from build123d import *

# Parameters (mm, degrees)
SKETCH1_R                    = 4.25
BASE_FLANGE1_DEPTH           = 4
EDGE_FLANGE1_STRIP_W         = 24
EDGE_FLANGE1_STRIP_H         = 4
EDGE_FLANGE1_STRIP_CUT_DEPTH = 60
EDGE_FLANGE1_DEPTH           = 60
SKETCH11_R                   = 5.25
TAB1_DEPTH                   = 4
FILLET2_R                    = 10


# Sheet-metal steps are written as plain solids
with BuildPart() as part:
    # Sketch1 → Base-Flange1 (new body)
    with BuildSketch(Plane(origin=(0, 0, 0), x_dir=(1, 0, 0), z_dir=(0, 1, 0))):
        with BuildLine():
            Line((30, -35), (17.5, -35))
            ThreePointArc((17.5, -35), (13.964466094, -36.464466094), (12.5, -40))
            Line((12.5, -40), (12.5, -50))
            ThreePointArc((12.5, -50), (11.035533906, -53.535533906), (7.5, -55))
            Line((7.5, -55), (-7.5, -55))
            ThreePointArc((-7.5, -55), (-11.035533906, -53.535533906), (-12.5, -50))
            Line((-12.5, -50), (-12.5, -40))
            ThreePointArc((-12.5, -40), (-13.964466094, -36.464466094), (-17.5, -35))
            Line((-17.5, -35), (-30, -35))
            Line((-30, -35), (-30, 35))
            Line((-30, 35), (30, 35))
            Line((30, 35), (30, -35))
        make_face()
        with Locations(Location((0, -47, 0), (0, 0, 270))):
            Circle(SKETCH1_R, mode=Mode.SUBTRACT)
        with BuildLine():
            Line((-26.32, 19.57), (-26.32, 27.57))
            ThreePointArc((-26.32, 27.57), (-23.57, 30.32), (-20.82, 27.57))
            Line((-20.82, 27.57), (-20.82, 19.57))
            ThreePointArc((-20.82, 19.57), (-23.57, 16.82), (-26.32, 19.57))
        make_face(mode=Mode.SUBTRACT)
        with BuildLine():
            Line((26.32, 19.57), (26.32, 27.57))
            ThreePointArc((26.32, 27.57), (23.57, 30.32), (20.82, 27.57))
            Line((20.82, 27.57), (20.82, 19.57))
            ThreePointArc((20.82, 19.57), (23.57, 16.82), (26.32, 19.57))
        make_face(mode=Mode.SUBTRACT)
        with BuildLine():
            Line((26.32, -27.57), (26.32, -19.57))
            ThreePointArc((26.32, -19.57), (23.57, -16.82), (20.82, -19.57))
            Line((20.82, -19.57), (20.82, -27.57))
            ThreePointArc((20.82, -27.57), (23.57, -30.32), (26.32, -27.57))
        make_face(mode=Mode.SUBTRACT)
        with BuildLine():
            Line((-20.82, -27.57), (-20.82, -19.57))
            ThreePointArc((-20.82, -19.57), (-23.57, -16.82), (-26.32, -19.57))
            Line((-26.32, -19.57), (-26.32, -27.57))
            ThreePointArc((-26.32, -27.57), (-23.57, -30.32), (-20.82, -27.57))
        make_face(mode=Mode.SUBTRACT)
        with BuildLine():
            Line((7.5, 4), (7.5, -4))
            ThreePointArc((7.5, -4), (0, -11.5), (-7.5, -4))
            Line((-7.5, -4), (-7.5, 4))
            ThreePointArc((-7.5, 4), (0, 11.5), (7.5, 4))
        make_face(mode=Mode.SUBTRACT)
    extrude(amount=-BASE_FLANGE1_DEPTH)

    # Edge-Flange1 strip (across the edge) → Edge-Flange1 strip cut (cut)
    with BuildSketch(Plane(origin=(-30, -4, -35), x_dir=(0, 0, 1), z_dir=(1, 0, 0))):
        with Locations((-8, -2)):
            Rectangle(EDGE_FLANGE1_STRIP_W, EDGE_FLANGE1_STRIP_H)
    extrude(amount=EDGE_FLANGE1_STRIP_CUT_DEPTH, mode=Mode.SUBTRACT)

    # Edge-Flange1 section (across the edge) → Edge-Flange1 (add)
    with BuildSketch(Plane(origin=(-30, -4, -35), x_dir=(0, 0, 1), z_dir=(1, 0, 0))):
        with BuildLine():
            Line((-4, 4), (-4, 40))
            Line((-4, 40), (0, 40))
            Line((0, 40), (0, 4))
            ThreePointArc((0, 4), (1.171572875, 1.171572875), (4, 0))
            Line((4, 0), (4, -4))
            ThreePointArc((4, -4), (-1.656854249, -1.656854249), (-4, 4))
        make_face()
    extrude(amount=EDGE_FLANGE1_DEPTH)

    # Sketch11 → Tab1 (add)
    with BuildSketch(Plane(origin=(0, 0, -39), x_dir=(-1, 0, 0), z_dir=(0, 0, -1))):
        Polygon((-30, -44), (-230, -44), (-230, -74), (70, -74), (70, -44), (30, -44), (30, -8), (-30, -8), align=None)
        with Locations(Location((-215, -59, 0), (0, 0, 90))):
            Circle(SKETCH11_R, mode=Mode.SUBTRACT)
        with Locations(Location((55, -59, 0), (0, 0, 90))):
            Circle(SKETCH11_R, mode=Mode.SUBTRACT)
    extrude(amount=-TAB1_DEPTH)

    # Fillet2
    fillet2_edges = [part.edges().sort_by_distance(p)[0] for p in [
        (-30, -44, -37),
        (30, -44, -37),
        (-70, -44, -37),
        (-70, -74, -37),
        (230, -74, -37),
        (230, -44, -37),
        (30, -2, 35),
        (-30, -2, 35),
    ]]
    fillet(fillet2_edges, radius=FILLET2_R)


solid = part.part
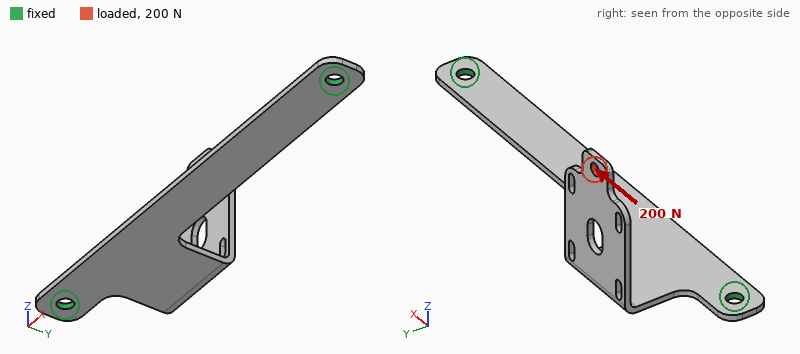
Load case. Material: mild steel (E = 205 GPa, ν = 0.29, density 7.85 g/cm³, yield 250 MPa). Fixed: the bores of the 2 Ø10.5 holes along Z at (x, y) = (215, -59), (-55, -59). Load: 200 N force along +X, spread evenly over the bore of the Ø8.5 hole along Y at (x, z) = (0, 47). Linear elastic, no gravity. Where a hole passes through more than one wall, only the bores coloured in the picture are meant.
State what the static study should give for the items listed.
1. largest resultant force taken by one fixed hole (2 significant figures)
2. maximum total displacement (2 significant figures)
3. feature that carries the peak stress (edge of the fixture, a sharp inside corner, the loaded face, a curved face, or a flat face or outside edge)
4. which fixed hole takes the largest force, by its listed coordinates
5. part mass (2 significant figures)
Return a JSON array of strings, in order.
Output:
["170 N", "1.3 mm", "a flat face or outside edge", "(-55, -59)", "480 g"]
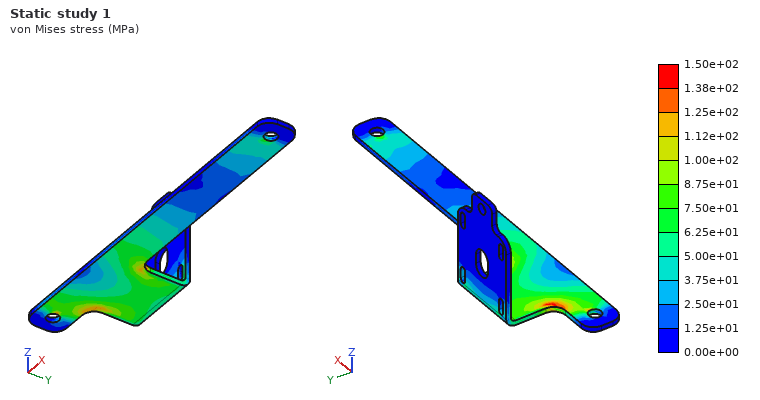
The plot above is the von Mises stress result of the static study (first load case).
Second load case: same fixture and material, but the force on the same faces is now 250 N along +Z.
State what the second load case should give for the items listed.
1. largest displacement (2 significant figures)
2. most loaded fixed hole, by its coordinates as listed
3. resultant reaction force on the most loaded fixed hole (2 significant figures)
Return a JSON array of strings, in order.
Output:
["1.4 mm", "(-55, -59)", "220 N"]
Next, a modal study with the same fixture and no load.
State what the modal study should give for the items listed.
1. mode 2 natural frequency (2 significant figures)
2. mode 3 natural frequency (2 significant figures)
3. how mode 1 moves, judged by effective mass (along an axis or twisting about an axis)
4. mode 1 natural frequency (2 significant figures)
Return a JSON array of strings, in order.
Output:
["240 Hz", "490 Hz", "along Z", "170 Hz"]
